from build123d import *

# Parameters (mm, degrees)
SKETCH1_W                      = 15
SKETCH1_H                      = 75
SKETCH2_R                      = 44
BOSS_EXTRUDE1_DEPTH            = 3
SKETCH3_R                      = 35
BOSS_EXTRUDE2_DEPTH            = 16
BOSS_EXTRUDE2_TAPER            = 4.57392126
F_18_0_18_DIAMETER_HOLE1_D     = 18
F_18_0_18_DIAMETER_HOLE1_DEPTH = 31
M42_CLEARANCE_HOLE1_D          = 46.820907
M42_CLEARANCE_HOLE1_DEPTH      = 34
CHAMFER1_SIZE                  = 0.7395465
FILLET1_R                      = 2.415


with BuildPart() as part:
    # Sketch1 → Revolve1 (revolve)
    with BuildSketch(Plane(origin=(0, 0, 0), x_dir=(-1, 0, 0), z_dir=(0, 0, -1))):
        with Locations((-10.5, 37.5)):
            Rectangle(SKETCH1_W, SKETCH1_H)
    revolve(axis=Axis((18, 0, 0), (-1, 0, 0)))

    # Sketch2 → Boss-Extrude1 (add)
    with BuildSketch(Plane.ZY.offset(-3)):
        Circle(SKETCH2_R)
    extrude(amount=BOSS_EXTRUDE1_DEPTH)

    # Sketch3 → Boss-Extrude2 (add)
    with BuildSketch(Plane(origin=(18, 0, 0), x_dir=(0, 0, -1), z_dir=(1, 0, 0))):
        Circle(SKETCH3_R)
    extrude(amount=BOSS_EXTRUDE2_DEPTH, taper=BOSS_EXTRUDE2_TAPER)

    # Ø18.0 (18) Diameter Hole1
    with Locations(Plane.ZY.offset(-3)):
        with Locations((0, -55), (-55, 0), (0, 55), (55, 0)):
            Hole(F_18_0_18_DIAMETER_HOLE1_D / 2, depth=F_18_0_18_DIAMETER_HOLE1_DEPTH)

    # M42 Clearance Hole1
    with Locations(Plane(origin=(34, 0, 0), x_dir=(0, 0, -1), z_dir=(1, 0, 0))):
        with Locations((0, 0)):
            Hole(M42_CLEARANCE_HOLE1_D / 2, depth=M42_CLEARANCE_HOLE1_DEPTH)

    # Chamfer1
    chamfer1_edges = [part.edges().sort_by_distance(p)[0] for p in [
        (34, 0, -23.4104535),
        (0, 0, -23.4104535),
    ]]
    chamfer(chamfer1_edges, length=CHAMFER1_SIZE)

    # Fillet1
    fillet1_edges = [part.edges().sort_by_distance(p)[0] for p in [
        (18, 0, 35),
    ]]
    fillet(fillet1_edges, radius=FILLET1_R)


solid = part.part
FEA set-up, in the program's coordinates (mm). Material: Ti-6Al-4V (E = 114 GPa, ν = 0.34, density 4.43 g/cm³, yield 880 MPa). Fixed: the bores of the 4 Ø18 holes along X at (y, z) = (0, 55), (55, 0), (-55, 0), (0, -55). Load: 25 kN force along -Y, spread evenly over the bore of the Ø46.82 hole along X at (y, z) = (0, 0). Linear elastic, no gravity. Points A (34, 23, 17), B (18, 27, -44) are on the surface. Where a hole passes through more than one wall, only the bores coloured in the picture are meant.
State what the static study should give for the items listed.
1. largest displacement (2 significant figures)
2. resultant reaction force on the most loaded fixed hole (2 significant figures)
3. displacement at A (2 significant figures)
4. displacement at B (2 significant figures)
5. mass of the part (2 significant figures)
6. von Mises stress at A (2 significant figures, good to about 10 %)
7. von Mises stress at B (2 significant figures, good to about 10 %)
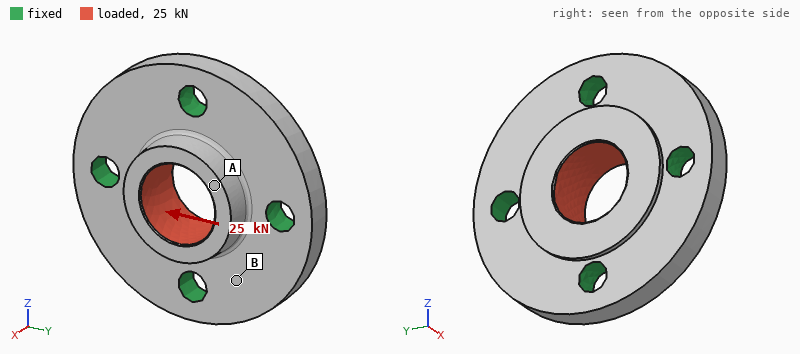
7.0 µm
7.8 kN
6.8 µm
1.8 µm
1.2 kg
8.6 MPa
3.8 MPa
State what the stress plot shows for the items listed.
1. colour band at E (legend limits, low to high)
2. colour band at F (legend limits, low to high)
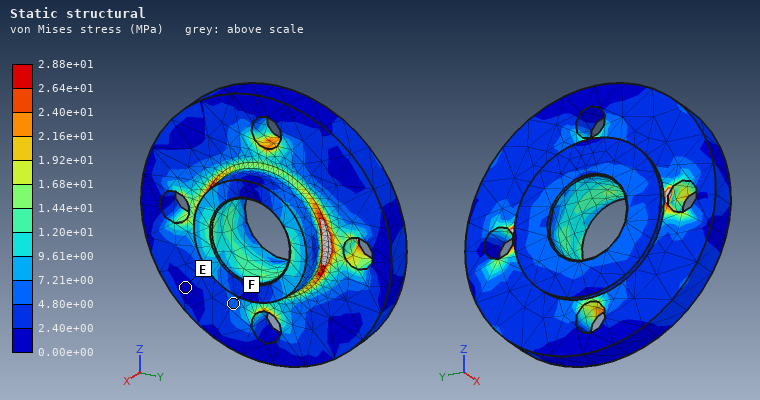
0.00e+00 to 2.40e+00 MPa
4.80e+00 to 7.21e+00 MPa
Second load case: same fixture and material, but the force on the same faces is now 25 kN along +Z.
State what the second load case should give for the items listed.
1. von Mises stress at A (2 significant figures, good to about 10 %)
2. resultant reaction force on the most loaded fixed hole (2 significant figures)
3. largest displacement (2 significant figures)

5.9 MPa
7.8 kN
7.0 µm
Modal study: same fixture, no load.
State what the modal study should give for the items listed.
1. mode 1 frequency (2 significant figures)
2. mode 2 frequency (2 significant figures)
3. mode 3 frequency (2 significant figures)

9300 Hz
9600 Hz
9600 Hz
